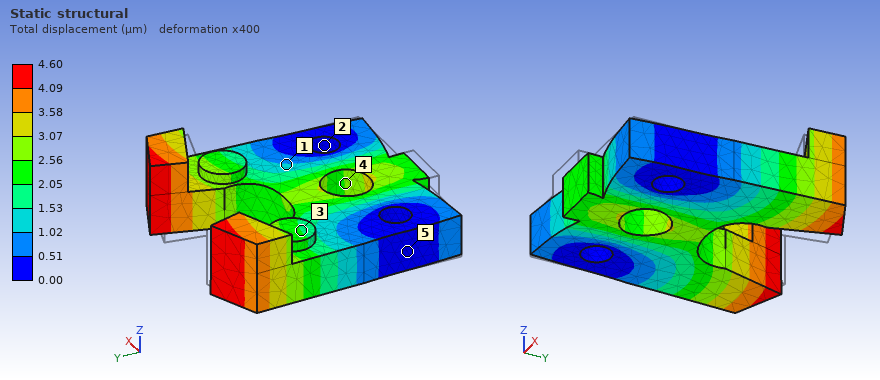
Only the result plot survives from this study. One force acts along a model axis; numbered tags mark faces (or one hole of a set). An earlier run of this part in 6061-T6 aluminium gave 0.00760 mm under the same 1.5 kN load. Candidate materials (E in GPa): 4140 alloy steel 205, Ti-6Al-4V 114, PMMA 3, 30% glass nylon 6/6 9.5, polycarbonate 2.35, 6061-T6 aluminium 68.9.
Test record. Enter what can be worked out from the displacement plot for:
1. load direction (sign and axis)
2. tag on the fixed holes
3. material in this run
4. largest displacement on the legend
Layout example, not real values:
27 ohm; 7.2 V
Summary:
+Y; 2; Ti-6Al-4V; 4.60 µm
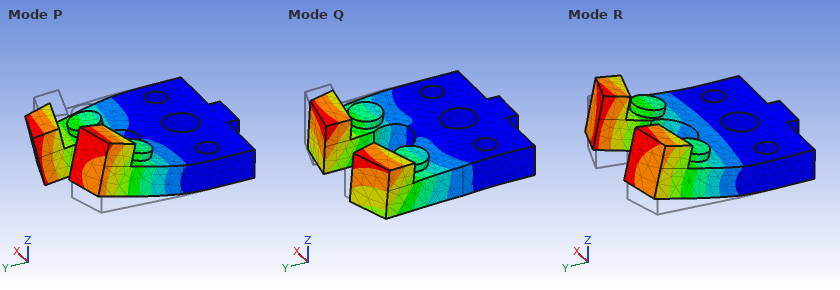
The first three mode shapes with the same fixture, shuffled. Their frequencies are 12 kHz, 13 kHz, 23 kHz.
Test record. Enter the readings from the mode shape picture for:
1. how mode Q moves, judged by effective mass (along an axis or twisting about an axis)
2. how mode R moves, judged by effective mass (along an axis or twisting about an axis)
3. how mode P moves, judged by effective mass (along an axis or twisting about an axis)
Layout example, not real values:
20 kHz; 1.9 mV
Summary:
along X; along Z; twisting about Y
